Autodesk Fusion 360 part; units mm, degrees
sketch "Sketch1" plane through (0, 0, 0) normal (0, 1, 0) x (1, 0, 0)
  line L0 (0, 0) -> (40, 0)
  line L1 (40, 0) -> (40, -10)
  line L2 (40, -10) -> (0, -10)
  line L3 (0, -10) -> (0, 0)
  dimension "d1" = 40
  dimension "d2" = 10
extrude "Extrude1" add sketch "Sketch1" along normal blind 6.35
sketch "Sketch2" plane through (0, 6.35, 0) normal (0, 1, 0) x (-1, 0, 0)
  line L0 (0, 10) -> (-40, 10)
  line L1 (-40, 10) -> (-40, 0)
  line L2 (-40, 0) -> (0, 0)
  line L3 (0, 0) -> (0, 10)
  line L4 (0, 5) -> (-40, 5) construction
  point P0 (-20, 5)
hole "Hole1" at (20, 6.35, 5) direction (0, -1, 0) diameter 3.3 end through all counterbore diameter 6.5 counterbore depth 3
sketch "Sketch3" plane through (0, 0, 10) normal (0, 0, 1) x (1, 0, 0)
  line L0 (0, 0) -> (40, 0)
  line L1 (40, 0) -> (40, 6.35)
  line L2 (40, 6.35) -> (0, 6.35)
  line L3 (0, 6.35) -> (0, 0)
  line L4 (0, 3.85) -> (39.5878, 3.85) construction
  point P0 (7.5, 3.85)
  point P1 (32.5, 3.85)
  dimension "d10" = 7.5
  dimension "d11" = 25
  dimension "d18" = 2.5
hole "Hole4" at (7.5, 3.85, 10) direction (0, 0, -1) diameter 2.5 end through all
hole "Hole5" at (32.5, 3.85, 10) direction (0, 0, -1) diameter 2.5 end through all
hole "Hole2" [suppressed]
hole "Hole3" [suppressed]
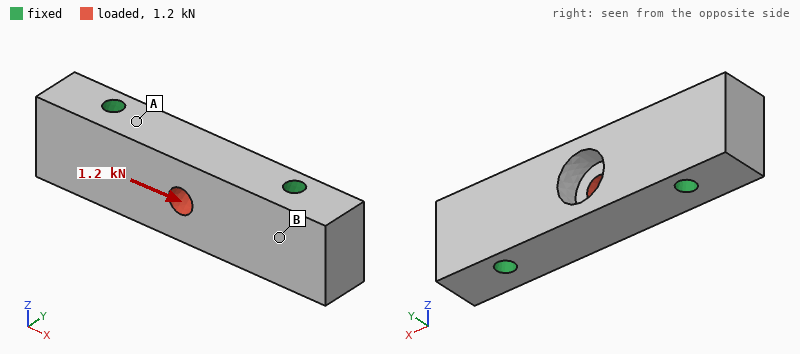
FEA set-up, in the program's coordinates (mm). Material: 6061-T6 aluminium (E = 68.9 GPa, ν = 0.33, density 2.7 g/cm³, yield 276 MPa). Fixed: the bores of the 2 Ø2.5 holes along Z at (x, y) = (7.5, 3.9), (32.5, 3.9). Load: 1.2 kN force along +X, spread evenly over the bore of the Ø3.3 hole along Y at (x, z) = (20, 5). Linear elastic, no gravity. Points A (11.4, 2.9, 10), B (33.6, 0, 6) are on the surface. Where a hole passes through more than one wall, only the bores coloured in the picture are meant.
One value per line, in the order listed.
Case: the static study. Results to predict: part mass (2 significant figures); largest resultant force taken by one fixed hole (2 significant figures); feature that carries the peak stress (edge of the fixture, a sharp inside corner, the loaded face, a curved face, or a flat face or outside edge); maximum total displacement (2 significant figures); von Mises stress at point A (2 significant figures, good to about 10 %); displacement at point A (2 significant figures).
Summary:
6.2 g
610 N
the loaded face
3.0 µm
12 MPa
0.61 µm
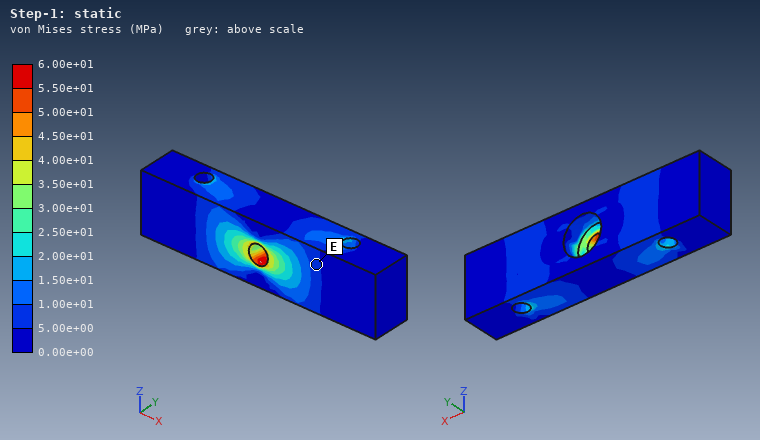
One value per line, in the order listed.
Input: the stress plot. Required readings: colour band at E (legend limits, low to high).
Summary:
5.00e+00 to 1.00e+01 MPa
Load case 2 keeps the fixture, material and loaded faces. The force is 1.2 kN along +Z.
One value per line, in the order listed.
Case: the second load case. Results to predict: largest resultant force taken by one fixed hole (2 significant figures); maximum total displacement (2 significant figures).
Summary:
600 N
11 µm
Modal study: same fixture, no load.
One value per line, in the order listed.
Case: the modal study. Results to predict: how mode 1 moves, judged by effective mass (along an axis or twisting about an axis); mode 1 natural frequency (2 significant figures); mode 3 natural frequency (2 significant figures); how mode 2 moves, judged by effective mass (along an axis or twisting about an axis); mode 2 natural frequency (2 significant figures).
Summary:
along Y
36 kHz
56 kHz
along Z
53 kHz
